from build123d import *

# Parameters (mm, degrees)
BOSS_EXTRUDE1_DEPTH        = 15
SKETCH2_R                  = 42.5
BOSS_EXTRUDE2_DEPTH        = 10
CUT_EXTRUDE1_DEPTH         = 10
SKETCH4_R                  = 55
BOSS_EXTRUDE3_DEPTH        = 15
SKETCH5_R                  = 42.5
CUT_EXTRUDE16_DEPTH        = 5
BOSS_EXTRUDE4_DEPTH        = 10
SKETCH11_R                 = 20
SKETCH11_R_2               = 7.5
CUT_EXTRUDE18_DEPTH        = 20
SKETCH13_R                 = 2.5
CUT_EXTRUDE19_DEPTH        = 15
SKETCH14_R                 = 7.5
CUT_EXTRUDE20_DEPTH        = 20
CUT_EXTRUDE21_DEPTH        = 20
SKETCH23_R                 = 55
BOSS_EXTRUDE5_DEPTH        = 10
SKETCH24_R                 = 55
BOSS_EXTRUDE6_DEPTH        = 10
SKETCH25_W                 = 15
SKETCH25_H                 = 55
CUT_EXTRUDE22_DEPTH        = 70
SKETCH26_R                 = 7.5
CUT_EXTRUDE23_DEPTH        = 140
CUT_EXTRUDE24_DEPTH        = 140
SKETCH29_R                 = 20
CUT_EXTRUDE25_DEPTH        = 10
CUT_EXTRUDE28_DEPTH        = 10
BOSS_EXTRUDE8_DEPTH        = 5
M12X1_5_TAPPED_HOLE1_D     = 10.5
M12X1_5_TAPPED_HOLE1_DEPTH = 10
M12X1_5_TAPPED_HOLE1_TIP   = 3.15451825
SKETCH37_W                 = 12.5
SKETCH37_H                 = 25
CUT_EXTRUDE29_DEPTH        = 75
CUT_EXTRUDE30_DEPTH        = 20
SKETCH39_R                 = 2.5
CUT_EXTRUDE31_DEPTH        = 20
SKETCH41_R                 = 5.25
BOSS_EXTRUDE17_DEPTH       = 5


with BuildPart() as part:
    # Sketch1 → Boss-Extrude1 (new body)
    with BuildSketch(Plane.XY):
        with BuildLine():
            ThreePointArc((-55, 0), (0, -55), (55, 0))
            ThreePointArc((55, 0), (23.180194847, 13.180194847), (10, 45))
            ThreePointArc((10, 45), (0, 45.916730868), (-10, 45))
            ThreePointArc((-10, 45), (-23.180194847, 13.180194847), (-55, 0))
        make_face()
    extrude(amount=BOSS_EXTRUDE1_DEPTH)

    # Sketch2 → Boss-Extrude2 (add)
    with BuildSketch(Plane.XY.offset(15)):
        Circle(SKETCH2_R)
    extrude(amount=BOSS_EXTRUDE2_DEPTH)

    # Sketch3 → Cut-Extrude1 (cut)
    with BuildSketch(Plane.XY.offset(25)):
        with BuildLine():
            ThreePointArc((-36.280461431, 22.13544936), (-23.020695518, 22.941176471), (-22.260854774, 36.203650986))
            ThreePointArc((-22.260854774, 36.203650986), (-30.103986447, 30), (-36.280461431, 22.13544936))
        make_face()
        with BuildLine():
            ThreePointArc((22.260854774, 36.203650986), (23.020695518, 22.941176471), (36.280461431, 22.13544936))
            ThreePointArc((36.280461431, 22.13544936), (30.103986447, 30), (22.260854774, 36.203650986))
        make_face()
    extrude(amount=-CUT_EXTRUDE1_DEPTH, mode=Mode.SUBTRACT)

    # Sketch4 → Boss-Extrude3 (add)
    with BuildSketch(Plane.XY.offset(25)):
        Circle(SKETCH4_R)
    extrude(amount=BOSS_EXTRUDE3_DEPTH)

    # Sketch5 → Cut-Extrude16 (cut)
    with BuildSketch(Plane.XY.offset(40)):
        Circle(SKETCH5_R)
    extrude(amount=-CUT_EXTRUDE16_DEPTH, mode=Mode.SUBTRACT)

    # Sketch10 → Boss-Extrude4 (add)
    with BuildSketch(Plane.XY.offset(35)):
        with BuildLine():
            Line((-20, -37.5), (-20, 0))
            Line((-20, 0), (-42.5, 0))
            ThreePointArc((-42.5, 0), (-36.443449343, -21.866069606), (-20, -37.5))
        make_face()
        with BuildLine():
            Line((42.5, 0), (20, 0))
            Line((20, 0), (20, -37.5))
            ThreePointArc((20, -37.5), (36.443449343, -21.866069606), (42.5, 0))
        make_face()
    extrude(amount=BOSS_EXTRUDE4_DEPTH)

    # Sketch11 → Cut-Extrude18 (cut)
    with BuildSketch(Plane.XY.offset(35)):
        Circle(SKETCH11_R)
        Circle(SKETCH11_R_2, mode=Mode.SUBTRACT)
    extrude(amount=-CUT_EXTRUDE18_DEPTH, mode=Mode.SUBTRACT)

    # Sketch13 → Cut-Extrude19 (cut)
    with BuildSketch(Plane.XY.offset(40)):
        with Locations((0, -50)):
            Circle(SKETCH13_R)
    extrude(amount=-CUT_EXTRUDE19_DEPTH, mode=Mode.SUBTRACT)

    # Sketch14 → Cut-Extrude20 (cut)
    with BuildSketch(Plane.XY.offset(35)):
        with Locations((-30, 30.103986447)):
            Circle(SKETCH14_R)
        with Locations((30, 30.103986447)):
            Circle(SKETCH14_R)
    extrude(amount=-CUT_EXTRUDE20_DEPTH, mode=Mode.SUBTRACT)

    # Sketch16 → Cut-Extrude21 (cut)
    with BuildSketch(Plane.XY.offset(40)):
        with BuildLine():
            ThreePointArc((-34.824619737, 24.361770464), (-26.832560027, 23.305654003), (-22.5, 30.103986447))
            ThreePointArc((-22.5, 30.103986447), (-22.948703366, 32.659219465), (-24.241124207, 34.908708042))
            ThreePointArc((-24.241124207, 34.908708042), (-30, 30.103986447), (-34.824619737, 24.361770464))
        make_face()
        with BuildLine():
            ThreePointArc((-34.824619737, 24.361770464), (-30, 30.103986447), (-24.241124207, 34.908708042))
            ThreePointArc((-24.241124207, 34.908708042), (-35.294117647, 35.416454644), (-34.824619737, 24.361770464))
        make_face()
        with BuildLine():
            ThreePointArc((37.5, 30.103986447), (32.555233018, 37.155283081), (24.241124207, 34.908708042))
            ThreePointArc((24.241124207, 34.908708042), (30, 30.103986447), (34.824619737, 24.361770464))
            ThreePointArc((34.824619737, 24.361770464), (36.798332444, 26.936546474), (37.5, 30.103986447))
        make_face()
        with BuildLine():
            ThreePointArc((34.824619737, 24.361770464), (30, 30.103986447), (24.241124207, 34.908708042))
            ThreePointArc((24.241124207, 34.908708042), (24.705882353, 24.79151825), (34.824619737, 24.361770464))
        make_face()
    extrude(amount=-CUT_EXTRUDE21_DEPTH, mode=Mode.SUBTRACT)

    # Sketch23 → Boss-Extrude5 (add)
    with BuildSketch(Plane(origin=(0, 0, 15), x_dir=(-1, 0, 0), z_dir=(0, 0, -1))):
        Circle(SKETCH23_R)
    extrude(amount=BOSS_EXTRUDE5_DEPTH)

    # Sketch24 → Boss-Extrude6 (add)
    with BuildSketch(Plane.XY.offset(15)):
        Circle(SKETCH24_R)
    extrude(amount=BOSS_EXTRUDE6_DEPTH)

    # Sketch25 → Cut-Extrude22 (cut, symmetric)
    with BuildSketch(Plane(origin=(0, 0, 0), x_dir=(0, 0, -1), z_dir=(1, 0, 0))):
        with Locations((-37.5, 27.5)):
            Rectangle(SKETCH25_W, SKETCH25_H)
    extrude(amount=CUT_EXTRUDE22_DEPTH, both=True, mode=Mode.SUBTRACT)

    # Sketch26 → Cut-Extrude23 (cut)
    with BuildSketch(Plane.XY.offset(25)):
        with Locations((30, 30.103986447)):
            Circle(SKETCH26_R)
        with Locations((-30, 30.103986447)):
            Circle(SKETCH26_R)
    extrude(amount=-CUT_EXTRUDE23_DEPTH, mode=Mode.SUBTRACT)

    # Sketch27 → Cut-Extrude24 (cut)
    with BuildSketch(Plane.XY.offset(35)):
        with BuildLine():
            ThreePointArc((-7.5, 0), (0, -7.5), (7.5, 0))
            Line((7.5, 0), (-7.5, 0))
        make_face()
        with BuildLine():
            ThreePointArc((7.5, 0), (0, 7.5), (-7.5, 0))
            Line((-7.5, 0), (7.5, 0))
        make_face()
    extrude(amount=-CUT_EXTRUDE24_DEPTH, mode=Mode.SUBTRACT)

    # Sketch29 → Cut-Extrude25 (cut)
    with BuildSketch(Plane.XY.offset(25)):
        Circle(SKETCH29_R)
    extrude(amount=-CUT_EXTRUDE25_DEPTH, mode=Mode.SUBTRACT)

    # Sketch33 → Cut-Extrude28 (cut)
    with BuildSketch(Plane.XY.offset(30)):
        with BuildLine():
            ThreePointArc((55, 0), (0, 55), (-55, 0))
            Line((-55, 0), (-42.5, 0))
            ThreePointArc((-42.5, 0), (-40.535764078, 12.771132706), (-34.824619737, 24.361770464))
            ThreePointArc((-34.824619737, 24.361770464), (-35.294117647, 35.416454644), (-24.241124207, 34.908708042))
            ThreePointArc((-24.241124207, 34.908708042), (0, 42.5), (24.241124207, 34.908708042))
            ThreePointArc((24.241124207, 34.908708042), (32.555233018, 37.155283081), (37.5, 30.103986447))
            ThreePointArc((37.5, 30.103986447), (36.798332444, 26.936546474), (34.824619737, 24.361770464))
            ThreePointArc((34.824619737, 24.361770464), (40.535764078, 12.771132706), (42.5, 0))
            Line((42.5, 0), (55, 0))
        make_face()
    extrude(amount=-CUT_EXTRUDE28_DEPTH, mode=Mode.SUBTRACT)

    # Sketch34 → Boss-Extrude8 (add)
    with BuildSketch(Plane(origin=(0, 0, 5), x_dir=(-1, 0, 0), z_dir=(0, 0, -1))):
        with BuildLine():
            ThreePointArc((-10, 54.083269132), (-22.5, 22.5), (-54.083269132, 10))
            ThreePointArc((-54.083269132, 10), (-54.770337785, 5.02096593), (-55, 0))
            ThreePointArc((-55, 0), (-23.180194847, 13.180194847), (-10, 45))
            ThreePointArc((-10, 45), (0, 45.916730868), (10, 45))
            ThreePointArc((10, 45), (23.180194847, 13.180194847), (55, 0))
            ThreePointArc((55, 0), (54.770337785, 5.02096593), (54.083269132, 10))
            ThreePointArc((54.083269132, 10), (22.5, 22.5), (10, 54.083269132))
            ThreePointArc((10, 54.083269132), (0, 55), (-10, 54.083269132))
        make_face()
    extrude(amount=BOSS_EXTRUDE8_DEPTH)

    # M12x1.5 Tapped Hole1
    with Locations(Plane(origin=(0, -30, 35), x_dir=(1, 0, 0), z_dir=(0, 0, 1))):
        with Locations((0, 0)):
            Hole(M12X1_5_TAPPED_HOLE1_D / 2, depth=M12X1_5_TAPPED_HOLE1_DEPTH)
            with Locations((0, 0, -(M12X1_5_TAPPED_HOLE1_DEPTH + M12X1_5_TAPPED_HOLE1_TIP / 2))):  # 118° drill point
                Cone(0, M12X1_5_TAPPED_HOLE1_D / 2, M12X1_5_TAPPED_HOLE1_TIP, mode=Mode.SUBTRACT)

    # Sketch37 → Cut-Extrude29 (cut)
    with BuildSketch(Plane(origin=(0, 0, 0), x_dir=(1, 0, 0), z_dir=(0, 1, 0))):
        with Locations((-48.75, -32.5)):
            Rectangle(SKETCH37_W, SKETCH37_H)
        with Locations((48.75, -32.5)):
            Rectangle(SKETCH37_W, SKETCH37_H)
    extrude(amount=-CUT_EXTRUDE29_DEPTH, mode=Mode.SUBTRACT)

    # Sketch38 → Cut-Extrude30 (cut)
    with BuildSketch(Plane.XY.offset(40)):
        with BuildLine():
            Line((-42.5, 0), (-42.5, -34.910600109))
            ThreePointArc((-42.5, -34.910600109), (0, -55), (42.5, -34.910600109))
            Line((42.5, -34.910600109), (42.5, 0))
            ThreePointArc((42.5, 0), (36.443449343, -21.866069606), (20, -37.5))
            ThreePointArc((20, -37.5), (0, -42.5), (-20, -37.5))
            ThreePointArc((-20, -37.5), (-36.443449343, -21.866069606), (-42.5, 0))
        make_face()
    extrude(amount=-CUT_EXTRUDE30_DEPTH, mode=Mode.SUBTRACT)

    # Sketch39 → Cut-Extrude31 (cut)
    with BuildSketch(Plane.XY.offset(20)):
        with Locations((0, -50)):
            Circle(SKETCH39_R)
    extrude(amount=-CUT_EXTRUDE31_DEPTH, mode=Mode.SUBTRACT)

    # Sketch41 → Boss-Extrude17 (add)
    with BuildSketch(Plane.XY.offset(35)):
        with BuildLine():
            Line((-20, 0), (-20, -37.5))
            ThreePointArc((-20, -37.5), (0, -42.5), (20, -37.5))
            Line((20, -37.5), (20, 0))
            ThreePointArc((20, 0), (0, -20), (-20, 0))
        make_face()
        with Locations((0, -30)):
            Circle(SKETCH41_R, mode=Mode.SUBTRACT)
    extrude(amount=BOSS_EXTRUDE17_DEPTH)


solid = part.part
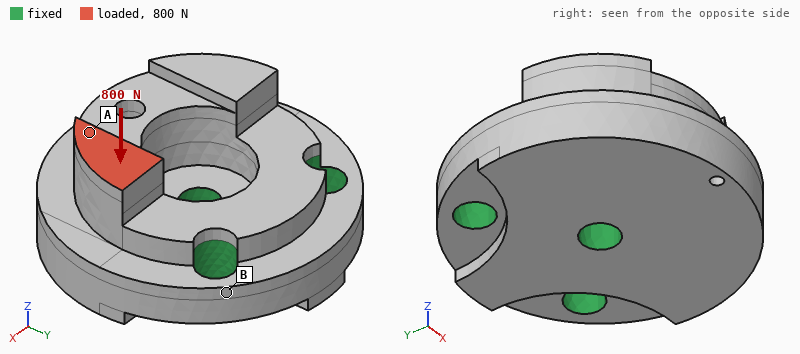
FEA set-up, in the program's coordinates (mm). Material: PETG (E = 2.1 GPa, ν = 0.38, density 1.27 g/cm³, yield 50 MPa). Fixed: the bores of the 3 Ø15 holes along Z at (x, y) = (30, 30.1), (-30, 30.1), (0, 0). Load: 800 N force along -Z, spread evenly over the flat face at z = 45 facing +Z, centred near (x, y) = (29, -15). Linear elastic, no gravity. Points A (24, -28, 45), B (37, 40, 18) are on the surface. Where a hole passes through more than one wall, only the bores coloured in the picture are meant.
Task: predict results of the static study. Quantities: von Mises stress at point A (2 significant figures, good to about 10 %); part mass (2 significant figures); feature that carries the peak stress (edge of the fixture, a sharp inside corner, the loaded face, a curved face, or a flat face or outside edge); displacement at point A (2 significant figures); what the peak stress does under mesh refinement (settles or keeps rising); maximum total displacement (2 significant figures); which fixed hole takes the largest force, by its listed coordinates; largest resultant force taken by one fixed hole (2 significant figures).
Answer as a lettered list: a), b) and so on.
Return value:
a) 1.2 MPa
b) 300 g
c) edge of the fixture
d) 0.12 mm
e) keeps rising
f) 0.14 mm
g) (0, 0)
h) 710 N
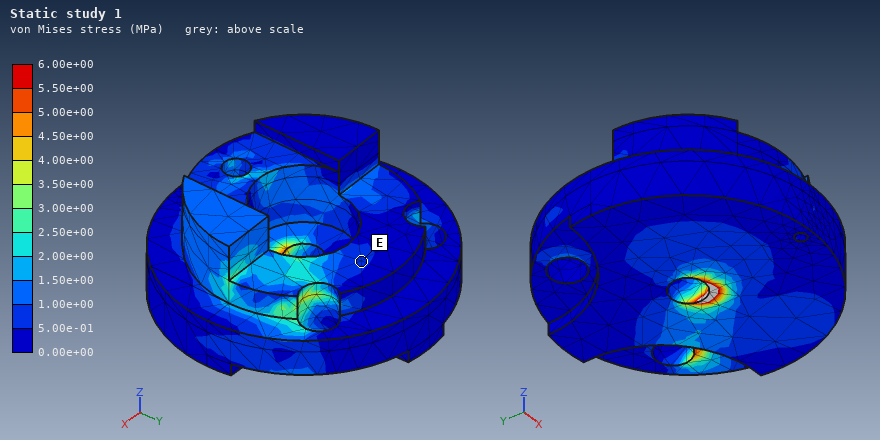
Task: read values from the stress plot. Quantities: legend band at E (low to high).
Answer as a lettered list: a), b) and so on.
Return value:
a) 5.00e-01 to 1.00e+00 MPa
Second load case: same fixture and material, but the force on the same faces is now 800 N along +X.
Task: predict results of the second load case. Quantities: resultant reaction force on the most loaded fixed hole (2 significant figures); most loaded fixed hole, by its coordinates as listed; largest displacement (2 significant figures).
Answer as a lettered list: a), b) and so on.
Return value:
a) 510 N
b) (0, 0)
c) 0.24 mm
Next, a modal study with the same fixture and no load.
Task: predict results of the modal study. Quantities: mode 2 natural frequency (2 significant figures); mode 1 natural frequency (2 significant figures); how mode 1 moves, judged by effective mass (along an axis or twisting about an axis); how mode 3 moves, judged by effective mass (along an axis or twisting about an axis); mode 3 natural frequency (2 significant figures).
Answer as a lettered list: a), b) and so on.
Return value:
a) 1500 Hz
b) 1300 Hz
c) along Z
d) along X
e) 2300 Hz
